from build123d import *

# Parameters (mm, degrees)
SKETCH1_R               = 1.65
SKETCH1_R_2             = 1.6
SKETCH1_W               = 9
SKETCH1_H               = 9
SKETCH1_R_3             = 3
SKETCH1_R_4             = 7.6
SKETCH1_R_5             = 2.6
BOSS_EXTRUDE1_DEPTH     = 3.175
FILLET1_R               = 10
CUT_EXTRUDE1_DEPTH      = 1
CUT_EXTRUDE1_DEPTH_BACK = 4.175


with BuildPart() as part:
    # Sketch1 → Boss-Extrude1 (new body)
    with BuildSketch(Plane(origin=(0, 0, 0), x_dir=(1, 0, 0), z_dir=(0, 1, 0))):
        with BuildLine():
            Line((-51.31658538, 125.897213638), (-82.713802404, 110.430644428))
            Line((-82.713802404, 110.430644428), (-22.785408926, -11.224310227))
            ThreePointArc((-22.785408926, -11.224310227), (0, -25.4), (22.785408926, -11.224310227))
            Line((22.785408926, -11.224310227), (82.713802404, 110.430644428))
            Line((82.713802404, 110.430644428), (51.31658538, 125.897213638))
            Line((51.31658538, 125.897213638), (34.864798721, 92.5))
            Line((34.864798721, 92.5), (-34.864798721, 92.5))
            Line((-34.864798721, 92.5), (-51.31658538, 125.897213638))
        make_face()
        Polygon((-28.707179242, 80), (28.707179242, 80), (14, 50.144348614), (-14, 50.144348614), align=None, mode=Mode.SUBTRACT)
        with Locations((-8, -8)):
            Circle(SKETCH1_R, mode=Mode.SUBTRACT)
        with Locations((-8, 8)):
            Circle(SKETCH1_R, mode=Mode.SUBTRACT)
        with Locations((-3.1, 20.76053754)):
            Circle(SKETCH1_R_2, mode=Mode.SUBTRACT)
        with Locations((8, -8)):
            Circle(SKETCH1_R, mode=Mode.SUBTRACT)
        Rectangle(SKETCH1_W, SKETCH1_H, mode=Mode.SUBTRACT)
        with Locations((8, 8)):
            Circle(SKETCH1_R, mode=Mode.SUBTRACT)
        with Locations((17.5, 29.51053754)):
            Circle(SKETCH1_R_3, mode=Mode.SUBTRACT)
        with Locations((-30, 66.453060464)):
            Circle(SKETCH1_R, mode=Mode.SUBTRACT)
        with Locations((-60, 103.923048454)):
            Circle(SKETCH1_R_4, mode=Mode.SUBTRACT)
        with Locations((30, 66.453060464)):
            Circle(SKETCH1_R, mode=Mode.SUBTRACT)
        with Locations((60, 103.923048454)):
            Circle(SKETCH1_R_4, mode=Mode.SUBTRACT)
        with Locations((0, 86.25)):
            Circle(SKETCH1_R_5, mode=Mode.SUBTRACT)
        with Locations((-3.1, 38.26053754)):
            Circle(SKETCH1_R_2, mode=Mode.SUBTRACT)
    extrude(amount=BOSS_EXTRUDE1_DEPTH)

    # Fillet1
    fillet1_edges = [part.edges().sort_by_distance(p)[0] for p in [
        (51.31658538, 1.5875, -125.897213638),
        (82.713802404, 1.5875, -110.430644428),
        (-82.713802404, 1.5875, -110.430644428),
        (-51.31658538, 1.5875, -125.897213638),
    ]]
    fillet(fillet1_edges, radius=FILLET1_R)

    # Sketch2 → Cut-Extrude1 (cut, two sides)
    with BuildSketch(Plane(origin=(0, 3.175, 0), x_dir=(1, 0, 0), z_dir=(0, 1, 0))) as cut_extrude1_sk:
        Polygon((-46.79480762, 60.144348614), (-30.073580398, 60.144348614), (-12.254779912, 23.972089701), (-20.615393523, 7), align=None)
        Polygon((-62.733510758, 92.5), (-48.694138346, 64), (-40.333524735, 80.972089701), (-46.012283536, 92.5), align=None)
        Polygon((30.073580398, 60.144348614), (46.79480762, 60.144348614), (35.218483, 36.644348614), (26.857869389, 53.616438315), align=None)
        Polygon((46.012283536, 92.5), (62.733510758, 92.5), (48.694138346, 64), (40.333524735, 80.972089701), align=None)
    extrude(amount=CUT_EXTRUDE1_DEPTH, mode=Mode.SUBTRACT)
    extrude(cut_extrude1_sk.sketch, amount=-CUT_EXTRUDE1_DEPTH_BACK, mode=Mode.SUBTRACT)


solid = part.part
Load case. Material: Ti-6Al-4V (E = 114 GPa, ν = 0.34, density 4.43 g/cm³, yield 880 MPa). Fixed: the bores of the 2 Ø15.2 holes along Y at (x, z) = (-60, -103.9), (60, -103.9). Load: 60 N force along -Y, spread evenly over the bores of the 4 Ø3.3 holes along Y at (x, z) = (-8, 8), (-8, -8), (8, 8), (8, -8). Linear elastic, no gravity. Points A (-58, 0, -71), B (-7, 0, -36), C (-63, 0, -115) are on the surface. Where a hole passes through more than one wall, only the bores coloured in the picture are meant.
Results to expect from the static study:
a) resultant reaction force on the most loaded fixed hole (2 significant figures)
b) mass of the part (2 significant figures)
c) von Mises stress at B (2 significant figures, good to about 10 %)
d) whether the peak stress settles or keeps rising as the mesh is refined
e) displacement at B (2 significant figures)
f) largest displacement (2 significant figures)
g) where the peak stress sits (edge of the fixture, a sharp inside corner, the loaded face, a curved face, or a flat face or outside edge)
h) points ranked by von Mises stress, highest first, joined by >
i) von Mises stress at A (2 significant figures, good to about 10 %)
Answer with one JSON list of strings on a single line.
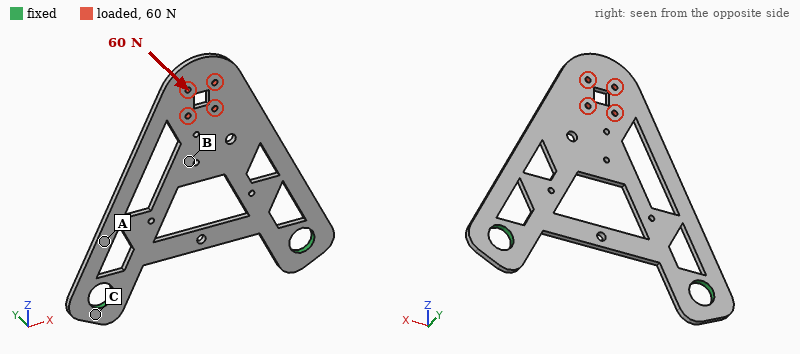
["31 N", "130 g", "21 MPa", "keeps rising", "0.81 mm", "2.1 mm", "a sharp inside corner", "A > B > C", "54 MPa"]
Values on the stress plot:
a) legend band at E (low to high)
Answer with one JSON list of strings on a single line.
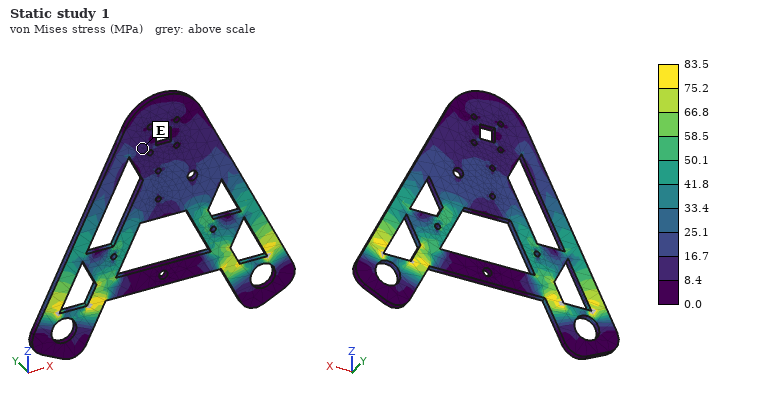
["8.4 to 16.7 MPa"]
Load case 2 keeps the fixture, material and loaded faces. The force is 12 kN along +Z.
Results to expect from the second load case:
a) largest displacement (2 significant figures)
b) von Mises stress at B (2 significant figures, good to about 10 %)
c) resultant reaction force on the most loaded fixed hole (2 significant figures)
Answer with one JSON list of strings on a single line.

["0.12 mm", "58 MPa", "6.8 kN"]
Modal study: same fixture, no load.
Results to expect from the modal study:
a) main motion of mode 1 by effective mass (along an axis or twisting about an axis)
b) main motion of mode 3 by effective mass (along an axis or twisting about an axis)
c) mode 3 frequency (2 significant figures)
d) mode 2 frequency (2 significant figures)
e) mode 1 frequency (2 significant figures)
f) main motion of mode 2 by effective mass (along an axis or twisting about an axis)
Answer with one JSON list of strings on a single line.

["along Y", "along Y", "870 Hz", "740 Hz", "160 Hz", "twisting about Z"]
